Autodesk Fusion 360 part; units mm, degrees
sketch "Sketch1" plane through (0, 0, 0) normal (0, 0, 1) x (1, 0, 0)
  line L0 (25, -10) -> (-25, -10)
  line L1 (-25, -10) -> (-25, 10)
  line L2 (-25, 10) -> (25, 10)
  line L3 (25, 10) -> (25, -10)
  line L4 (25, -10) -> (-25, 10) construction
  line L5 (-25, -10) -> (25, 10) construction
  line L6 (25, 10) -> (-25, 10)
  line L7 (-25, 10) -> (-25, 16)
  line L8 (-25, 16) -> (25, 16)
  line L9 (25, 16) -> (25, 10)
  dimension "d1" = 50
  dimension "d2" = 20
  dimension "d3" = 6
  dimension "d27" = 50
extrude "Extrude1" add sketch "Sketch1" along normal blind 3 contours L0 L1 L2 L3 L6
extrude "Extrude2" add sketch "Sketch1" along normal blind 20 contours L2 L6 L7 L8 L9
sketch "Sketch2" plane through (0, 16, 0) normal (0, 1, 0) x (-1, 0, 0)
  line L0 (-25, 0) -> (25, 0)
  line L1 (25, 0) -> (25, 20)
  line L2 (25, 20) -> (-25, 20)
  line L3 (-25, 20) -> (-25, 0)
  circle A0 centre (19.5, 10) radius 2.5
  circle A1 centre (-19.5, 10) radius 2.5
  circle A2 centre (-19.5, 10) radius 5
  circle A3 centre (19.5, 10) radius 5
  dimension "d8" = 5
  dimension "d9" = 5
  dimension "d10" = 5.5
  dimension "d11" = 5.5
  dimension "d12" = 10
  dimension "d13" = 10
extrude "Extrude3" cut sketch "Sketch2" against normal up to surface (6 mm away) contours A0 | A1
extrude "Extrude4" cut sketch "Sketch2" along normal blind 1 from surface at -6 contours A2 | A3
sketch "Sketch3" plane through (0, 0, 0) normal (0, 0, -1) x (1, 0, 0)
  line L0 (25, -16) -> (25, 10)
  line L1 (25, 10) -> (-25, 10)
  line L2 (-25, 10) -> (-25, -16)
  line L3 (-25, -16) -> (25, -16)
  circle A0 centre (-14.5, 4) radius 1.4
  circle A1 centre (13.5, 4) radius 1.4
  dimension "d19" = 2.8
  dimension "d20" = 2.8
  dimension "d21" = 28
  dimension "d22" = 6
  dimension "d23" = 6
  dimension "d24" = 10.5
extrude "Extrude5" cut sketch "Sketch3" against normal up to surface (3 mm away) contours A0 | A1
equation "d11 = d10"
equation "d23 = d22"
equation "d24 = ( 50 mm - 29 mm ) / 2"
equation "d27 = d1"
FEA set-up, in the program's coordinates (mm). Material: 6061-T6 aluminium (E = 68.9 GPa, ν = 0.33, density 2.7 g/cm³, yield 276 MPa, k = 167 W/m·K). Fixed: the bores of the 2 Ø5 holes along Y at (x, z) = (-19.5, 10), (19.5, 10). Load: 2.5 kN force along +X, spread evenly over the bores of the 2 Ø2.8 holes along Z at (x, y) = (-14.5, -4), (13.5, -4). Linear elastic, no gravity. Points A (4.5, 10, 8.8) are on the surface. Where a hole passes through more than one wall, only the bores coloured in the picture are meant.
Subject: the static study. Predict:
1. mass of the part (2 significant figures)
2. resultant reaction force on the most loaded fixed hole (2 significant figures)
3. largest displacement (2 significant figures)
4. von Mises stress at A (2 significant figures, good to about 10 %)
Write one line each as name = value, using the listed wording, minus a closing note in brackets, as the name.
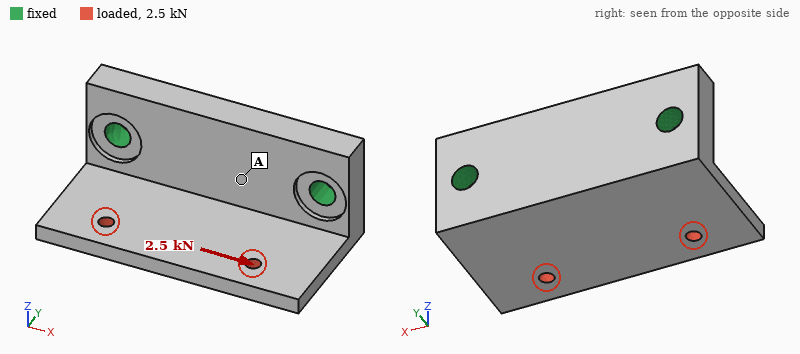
mass of the part = 23 g
resultant reaction force on the most loaded fixed hole = 1.7 kN
largest displacement = 54 µm
von Mises stress at A = 24 MPa
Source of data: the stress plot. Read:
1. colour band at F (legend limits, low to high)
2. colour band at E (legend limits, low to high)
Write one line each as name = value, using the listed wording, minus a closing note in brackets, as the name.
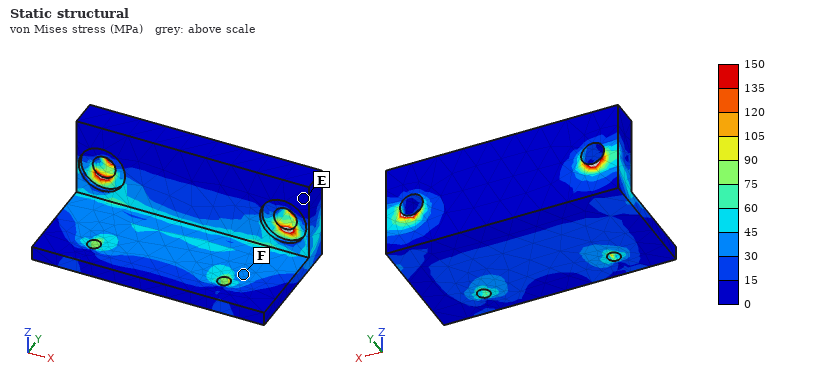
colour band at F = 30 to 45 MPa
colour band at E = 0 to 15 MPa
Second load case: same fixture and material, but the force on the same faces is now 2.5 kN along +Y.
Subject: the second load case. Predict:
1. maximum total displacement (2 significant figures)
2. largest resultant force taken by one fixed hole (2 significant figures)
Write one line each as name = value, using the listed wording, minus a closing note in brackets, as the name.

maximum total displacement = 71 µm
largest resultant force taken by one fixed hole = 1.3 kN
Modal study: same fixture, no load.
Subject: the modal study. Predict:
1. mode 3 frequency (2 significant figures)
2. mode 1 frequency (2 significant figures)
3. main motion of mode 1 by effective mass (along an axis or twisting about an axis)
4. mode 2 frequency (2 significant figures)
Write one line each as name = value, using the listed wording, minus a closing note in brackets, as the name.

mode 3 frequency = 12 kHz
mode 1 frequency = 4700 Hz
main motion of mode 1 by effective mass = along Z
mode 2 frequency = 6900 Hz
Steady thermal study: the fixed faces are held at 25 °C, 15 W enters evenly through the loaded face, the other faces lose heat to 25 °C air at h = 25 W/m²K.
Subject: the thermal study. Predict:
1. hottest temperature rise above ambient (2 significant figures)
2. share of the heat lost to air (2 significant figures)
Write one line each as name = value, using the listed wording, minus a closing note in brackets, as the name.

hottest temperature rise above ambient = 16 K
share of the heat lost to air = 4.6 %
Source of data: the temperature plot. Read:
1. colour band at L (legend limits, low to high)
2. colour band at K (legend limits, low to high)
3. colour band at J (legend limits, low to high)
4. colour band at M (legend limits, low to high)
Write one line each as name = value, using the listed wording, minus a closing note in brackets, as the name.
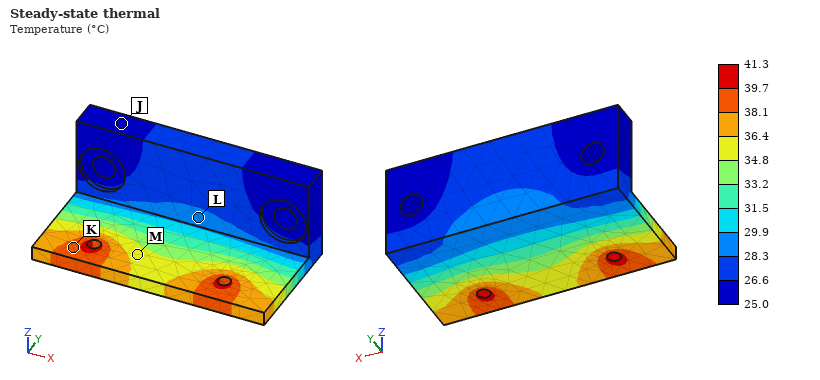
colour band at L = 28.3 to 29.9 °C
colour band at K = 38.1 to 39.7 °C
colour band at J = 25.0 to 26.6 °C
colour band at M = 34.8 to 36.4 °C
